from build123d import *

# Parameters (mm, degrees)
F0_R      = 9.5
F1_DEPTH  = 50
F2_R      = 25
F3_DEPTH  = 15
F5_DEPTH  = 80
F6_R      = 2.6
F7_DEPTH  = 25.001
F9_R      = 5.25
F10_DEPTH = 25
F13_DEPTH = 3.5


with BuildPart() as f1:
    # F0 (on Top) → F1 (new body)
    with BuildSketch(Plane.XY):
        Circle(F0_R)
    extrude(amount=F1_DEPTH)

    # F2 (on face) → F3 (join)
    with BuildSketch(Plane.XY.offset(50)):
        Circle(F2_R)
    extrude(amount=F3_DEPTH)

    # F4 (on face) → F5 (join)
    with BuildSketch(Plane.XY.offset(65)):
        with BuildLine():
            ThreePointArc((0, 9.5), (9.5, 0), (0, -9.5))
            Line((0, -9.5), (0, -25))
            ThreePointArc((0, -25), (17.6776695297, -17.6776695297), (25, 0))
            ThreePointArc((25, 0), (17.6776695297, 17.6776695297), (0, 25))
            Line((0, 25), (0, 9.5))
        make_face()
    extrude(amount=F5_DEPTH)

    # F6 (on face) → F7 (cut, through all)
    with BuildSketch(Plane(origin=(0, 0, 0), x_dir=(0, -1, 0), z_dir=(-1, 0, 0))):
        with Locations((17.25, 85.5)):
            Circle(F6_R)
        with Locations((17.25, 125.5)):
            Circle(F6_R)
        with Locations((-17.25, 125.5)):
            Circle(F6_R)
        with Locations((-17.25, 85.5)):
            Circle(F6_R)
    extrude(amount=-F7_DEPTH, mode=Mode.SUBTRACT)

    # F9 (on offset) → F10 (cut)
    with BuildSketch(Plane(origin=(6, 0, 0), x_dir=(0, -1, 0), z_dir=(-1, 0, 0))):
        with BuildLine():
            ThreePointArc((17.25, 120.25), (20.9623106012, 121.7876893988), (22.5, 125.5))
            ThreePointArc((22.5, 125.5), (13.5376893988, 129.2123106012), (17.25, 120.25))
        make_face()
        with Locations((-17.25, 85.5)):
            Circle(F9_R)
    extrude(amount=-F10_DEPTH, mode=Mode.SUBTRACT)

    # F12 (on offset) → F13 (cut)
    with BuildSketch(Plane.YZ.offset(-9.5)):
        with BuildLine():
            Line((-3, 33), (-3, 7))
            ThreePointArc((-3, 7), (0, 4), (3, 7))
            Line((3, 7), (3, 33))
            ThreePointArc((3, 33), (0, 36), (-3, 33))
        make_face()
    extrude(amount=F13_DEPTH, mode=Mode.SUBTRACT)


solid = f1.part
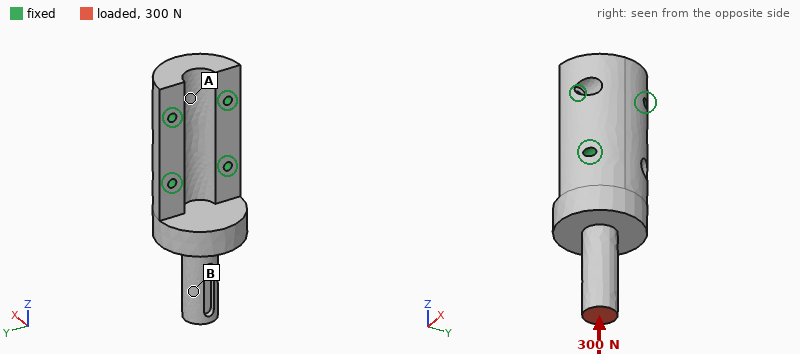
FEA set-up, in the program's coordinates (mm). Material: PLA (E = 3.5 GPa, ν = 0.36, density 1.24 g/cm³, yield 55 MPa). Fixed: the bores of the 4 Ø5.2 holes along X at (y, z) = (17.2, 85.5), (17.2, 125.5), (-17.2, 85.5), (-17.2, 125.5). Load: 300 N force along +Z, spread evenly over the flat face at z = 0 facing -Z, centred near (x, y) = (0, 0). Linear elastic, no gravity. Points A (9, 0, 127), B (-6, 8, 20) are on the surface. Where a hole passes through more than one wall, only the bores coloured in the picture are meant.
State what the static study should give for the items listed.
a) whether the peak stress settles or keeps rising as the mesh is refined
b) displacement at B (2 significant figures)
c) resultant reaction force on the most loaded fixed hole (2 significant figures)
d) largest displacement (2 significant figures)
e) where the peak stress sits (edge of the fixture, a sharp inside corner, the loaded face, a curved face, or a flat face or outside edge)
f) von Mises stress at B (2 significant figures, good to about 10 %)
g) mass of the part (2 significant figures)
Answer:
keeps rising
0.069 mm
150 N
0.10 mm
edge of the fixture
1.4 MPa
130 g
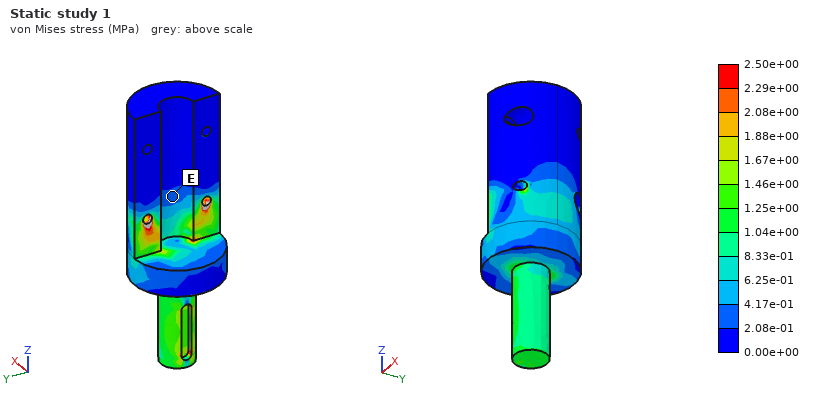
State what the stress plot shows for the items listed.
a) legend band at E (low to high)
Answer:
2.08e-01 to 4.17e-01 MPa
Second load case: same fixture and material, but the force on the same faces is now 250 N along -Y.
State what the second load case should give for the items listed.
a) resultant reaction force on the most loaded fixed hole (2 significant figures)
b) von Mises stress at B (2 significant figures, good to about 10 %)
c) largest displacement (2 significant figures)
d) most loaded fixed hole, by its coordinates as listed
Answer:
590 N
6.0 MPa
0.75 mm
(-17.2, 85.5)
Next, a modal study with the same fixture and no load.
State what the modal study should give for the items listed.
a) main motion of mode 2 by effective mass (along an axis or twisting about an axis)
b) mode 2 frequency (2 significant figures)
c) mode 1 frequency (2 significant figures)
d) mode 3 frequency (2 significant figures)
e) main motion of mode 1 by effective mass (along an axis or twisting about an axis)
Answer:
along Y
1300 Hz
870 Hz
2100 Hz
along X
